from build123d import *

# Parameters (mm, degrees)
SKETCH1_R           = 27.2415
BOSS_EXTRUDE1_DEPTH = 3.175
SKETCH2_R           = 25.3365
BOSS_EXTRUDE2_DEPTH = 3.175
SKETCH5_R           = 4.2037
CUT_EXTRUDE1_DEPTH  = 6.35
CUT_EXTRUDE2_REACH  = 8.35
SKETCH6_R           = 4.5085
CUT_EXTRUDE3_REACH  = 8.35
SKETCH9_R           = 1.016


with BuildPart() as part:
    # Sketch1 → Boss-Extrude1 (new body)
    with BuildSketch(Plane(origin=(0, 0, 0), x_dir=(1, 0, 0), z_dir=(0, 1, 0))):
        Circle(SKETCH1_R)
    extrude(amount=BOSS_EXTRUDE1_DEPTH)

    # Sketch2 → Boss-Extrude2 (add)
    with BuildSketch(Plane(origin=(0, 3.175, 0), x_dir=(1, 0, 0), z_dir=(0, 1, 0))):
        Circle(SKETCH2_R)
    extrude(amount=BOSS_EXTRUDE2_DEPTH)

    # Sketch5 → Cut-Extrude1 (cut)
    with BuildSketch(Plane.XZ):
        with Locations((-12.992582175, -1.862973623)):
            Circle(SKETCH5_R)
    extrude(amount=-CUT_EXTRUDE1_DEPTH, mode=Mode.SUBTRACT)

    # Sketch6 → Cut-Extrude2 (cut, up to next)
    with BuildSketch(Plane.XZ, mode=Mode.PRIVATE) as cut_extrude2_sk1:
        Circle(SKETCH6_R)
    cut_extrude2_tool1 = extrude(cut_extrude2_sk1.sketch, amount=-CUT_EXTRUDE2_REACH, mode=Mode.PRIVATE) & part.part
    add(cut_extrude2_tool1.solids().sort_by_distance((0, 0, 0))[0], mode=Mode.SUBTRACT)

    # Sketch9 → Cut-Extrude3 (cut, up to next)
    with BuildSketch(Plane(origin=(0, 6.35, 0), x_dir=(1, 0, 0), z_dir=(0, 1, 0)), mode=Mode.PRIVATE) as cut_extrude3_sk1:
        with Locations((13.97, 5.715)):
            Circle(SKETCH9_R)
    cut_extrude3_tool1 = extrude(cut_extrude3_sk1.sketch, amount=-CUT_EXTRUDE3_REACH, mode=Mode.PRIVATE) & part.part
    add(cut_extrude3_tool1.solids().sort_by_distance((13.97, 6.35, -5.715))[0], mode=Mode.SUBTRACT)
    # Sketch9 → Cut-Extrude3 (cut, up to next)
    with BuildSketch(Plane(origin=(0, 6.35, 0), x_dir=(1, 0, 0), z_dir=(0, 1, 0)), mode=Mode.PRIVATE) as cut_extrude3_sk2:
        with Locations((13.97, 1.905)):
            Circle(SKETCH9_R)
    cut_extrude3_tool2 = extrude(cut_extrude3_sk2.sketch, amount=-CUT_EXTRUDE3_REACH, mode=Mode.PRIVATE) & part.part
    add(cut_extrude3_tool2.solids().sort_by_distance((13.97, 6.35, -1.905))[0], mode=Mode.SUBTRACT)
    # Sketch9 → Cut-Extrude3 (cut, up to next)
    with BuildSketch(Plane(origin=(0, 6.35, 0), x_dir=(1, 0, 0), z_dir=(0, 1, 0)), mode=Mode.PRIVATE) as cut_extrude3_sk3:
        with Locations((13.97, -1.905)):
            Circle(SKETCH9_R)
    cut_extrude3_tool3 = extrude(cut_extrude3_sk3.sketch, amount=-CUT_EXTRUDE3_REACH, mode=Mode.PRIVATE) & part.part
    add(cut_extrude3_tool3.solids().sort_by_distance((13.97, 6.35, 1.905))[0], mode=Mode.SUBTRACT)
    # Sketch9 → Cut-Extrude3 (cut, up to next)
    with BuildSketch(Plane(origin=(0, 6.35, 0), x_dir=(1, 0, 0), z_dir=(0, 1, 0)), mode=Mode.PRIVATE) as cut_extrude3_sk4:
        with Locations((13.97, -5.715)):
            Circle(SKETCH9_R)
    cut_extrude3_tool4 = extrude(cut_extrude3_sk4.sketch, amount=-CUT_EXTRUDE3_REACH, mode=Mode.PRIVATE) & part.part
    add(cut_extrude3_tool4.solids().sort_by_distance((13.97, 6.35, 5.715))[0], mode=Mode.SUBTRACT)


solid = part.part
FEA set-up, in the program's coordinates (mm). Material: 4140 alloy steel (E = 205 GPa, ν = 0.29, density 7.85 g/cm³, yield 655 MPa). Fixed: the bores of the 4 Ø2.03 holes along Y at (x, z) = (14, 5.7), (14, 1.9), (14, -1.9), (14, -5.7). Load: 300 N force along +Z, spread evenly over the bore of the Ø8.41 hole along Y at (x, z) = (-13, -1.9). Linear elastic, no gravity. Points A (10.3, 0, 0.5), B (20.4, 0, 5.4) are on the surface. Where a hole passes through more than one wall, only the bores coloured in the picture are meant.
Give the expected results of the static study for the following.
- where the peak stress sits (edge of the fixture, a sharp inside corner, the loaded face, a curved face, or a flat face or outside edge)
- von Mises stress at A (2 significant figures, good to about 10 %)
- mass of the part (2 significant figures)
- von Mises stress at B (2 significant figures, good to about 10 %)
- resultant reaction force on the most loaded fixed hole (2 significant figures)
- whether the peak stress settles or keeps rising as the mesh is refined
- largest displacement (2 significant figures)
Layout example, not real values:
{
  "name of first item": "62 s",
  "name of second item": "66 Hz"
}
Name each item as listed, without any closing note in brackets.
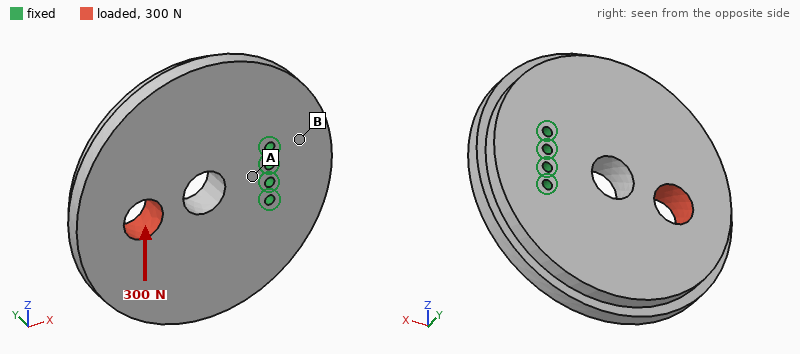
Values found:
{
  "where the peak stress sits": "edge of the fixture",
  "von Mises stress at A": "12 MPa",
  "mass of the part": "100 g",
  "von Mises stress at B": "4.5 MPa",
  "resultant reaction force on the most loaded fixed hole": "580 N",
  "whether the peak stress settles or keeps rising as the mesh is refined": "keeps rising",
  "largest displacement": "3.8 µm"
}
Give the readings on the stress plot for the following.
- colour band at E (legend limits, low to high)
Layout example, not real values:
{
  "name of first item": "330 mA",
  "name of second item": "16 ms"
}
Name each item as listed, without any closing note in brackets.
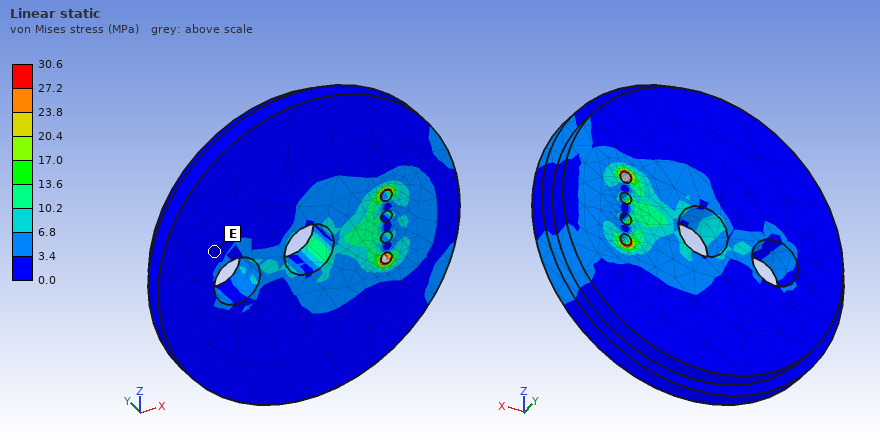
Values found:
{
  "colour band at E": "0.0 to 3.4 MPa"
}
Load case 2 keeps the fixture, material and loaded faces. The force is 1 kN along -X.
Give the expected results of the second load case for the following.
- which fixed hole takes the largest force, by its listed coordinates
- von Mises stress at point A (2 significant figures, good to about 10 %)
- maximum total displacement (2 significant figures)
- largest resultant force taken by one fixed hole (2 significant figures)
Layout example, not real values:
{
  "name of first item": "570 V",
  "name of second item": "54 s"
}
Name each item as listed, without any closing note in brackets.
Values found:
{
  "which fixed hole takes the largest force, by its listed coordinates": "(14, -5.7)",
  "von Mises stress at point A": "3.0 MPa",
  "maximum total displacement": "1.6 µm",
  "largest resultant force taken by one fixed hole": "510 N"
}
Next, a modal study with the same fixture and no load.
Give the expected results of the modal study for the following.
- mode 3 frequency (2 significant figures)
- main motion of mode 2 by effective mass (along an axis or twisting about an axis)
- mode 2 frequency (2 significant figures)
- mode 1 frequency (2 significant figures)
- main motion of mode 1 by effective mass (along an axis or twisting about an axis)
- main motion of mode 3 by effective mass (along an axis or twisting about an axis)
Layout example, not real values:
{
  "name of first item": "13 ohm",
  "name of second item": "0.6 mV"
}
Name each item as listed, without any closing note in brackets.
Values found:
{
  "mode 3 frequency": "6600 Hz",
  "main motion of mode 2 by effective mass": "twisting about X",
  "mode 2 frequency": "5500 Hz",
  "mode 1 frequency": "3200 Hz",
  "main motion of mode 1 by effective mass": "along Y",
  "main motion of mode 3 by effective mass": "along Z"
}
